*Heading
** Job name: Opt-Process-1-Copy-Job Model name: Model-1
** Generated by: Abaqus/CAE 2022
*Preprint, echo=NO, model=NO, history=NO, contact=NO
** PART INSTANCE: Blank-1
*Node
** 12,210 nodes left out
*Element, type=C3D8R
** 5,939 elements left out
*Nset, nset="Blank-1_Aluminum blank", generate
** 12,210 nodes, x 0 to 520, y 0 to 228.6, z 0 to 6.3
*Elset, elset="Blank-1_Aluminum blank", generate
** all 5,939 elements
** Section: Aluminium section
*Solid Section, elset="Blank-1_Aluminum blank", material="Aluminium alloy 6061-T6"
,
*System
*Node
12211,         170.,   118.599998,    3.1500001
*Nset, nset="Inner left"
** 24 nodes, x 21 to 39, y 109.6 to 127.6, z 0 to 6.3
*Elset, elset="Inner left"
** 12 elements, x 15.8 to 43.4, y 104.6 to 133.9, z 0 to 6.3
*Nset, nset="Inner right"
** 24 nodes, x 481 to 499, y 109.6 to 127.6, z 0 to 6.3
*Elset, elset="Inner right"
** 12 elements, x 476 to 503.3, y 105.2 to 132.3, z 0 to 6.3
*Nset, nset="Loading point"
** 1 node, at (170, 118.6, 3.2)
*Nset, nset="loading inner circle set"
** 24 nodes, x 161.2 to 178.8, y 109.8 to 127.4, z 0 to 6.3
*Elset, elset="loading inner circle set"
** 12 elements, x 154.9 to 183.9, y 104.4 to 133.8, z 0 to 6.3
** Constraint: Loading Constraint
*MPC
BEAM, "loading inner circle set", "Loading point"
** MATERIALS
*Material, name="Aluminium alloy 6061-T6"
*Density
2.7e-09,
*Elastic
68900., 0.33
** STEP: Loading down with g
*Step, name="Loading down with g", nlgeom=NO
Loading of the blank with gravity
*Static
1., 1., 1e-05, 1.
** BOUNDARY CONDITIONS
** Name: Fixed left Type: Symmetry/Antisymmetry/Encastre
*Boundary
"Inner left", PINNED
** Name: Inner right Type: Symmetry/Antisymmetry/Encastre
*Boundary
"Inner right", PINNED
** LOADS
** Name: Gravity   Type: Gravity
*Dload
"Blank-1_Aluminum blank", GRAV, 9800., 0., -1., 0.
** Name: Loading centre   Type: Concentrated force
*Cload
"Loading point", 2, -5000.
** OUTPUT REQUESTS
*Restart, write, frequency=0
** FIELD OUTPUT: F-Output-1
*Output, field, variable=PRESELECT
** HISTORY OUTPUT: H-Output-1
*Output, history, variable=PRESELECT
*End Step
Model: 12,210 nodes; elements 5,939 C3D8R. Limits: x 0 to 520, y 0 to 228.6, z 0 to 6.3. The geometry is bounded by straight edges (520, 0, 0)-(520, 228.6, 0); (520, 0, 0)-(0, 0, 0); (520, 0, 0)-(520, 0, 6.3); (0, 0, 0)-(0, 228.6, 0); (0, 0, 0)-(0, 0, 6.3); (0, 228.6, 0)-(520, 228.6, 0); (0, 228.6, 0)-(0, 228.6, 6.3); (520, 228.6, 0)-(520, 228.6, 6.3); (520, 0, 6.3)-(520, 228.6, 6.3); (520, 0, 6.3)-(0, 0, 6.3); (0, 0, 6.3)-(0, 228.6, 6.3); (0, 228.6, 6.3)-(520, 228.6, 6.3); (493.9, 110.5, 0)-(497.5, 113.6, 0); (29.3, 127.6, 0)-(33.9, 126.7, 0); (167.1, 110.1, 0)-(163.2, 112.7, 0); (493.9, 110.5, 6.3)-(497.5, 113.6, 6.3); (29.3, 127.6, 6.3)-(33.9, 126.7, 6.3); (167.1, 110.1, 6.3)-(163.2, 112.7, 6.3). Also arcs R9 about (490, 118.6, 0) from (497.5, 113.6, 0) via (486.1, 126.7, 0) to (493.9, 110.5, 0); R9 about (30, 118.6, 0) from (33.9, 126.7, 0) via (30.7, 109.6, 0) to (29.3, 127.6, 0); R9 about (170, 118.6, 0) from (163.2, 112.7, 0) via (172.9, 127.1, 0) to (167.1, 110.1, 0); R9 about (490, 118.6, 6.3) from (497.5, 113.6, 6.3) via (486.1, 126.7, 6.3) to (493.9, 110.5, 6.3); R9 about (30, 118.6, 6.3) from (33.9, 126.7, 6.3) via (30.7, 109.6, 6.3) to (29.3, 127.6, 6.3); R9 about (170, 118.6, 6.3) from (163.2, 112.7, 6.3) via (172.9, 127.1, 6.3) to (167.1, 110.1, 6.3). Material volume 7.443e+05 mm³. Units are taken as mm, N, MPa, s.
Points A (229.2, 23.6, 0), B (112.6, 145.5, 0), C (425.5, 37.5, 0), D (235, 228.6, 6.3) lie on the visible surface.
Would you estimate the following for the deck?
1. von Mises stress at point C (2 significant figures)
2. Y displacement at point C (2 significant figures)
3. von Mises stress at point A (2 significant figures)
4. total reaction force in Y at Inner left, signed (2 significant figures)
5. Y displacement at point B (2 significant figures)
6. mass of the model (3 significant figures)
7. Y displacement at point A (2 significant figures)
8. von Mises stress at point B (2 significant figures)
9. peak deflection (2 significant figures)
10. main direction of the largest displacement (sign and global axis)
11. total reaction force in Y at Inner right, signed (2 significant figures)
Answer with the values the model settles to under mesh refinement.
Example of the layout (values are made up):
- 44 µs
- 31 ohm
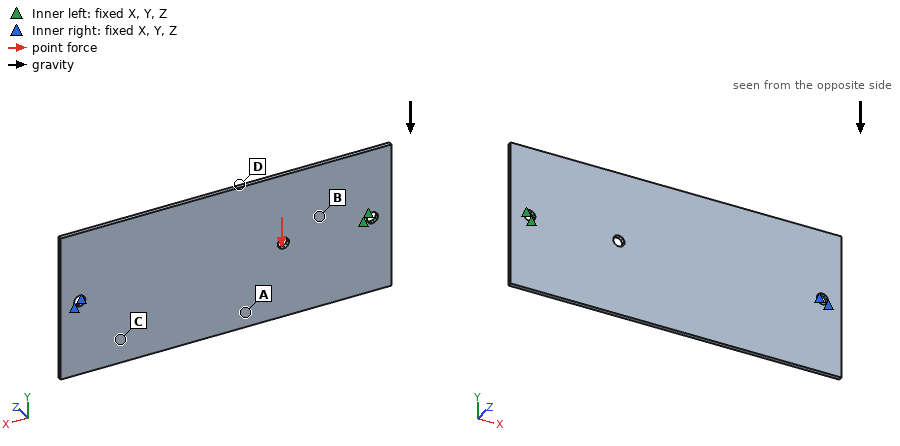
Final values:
- 1.8 MPa
- -0.011 mm
- 5.9 MPa
- 3500 N
- -0.022 mm
- 2.01 kg
- -0.031 mm
- 5.5 MPa
- 0.037 mm
- -Y
- 1500 N
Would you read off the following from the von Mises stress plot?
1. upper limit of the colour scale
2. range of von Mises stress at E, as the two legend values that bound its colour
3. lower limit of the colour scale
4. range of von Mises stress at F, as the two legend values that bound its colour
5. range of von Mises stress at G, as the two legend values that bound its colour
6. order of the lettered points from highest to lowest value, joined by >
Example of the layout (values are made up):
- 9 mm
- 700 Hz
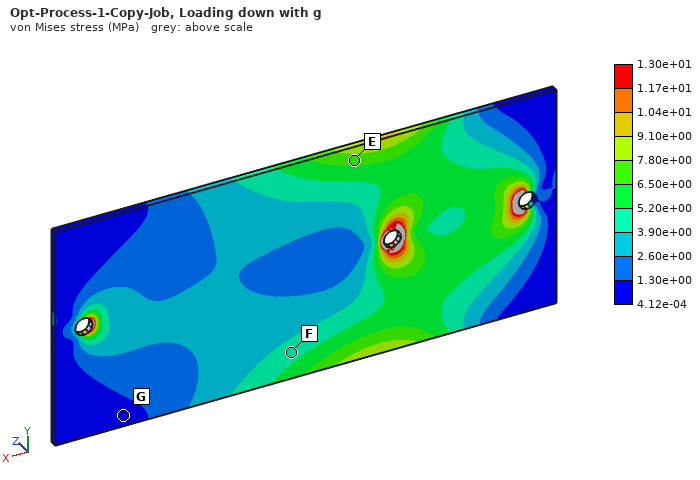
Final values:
- 1.30e+01 MPa
- 6.50e+00 to 7.80e+00 MPa
- 4.12e-04 MPa
- 3.90e+00 to 5.20e+00 MPa
- 4.12e-04 to 1.30e+00 MPa
- E > F > G
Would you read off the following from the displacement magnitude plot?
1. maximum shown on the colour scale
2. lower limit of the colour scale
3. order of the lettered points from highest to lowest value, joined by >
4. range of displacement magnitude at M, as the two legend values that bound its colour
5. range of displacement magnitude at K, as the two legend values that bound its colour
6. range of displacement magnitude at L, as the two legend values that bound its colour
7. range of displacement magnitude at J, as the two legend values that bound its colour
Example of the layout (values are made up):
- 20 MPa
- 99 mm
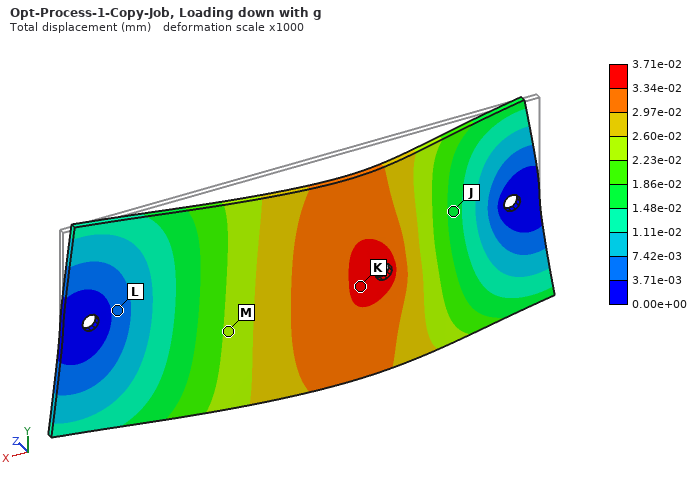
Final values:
- 3.71e-02 mm
- 0.00e+00 mm
- K > M > J > L
- 2.23e-02 to 2.60e-02 mm
- 3.34e-02 to 3.71e-02 mm
- 3.71e-03 to 7.42e-03 mm
- 1.48e-02 to 1.86e-02 mm
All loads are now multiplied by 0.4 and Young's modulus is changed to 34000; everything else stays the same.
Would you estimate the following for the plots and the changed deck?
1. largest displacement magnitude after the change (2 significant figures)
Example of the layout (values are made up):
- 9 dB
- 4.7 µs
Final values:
- 0.030 mm
